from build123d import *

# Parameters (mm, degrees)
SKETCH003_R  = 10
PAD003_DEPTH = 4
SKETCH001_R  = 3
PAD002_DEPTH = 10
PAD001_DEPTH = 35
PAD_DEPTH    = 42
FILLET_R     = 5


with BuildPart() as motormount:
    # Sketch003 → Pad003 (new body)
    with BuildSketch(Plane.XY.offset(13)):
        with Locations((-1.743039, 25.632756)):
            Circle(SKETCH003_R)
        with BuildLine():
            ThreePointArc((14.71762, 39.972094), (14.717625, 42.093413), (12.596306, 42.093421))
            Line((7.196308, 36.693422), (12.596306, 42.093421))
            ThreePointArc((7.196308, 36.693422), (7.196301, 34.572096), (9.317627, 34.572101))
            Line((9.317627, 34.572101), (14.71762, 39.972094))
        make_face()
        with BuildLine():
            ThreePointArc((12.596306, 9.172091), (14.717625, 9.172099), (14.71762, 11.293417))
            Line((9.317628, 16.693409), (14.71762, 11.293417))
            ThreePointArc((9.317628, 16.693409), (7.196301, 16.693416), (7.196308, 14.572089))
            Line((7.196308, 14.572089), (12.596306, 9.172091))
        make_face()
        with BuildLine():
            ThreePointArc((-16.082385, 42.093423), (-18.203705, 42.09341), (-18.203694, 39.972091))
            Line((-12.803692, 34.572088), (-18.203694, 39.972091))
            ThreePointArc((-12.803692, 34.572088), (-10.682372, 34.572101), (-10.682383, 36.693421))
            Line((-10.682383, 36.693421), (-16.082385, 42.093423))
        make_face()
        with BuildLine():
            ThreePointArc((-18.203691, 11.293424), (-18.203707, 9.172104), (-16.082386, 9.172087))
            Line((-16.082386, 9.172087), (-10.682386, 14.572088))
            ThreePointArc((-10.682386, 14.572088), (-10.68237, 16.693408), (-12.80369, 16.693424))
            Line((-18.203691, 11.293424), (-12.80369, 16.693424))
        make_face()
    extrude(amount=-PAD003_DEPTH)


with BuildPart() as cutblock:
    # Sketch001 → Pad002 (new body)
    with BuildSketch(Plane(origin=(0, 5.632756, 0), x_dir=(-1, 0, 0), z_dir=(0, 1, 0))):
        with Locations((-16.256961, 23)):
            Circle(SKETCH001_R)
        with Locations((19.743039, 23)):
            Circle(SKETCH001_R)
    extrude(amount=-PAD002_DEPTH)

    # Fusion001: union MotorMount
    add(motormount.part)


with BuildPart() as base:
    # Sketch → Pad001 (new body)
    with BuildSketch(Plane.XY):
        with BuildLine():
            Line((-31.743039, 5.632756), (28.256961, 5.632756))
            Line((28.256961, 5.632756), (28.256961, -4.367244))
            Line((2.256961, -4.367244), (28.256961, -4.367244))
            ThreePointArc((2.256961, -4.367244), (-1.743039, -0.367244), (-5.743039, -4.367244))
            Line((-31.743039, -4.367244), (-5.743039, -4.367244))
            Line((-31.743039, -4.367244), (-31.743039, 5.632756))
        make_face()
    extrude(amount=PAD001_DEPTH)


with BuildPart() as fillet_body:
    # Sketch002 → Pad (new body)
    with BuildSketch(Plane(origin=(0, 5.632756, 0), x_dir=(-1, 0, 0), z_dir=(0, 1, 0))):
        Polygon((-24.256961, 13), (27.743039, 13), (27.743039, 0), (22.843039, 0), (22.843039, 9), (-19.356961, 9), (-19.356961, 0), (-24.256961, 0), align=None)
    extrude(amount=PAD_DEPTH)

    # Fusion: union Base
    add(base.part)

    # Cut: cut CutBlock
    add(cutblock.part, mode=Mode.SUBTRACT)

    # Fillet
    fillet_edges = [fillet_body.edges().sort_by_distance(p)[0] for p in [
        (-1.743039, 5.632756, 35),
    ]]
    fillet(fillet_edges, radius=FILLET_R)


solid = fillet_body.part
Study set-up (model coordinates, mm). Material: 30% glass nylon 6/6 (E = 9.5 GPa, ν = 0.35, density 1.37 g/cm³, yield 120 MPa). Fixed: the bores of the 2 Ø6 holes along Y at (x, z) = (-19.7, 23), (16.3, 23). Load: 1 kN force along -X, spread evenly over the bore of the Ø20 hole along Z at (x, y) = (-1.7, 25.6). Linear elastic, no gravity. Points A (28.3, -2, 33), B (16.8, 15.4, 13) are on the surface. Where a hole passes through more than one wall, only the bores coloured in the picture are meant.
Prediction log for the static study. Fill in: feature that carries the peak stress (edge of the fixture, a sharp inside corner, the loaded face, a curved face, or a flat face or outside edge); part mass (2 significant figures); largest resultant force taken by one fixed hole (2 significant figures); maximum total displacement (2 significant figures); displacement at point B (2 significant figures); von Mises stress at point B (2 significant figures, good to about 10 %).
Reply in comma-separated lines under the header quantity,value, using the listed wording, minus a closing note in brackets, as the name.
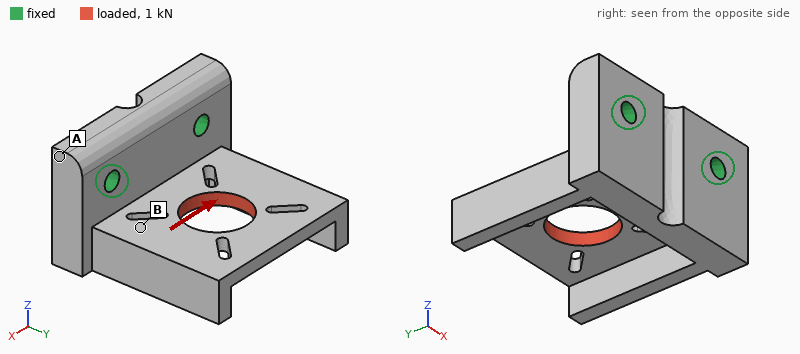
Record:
quantity,value
feature that carries the peak stress,a curved face
part mass,41 g
largest resultant force taken by one fixed hole,810 N
maximum total displacement,0.17 mm
displacement at point B,0.060 mm
von Mises stress at point B,8.7 MPa
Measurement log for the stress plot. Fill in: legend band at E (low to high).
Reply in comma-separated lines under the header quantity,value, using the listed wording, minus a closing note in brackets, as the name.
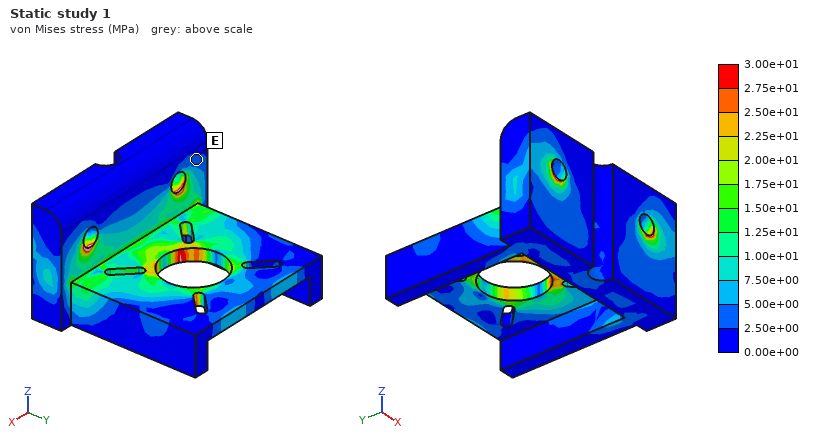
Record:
quantity,value
legend band at E,2.50e+00 to 5.00e+00 MPa
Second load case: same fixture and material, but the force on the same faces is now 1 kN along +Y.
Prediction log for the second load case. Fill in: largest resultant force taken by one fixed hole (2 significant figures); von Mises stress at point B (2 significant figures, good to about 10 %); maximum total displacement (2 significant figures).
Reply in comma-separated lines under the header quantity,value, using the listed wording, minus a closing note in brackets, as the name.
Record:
quantity,value
largest resultant force taken by one fixed hole,510 N
von Mises stress at point B,8.1 MPa
maximum total displacement,81 µm
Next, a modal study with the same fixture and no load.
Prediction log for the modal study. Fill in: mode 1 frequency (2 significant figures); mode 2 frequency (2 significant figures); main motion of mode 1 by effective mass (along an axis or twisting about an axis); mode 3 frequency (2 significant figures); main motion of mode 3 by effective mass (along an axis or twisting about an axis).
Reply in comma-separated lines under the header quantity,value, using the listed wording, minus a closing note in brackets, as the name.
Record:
quantity,value
mode 1 frequency,1500 Hz
mode 2 frequency,2100 Hz
main motion of mode 1 by effective mass,along Z
mode 3 frequency,3300 Hz
main motion of mode 3 by effective mass,along X
